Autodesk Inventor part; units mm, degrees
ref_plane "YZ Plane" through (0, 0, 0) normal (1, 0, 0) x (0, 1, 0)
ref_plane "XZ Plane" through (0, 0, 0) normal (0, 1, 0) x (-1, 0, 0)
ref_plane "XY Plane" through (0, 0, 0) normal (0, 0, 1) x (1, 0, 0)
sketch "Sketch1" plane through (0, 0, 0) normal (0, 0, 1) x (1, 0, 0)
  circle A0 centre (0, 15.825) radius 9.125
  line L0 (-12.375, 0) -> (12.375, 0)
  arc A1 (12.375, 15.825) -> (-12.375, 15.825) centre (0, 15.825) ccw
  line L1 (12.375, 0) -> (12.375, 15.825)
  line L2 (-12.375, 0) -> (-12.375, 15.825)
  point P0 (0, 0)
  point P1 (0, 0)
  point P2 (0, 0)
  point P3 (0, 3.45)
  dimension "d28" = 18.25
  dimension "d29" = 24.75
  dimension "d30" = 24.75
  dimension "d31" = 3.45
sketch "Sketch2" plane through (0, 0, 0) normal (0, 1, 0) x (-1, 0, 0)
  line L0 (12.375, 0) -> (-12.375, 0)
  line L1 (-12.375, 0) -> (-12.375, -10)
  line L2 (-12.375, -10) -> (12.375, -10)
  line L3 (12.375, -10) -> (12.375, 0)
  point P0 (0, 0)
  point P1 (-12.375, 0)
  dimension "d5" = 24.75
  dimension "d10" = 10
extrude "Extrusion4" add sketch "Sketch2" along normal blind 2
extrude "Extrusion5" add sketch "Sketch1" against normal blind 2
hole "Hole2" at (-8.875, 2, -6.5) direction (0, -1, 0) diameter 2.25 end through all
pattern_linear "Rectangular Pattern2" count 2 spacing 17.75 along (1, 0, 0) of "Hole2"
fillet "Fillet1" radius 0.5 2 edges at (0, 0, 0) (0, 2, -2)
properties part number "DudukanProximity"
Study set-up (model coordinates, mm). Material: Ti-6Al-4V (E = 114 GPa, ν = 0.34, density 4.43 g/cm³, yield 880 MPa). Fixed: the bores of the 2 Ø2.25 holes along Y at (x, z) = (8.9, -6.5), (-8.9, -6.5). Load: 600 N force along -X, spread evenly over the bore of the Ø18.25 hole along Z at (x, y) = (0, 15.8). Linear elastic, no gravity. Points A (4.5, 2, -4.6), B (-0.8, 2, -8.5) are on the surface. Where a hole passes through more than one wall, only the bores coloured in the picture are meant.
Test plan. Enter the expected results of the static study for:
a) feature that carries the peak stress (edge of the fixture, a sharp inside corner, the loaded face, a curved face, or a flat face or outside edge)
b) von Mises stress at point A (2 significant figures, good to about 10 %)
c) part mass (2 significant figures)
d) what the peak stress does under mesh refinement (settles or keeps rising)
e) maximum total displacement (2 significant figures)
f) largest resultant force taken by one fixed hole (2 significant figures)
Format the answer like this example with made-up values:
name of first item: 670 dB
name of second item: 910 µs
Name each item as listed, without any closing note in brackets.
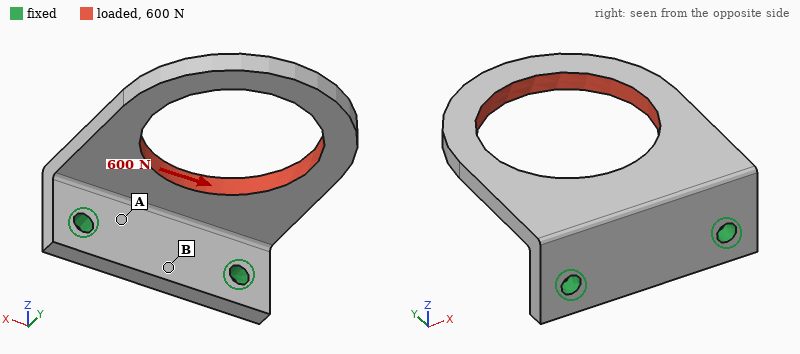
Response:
feature that carries the peak stress: edge of the fixture
von Mises stress at point A: 93 MPa
part mass: 5.0 g
what the peak stress does under mesh refinement: keeps rising
maximum total displacement: 0.15 mm
largest resultant force taken by one fixed hole: 580 N
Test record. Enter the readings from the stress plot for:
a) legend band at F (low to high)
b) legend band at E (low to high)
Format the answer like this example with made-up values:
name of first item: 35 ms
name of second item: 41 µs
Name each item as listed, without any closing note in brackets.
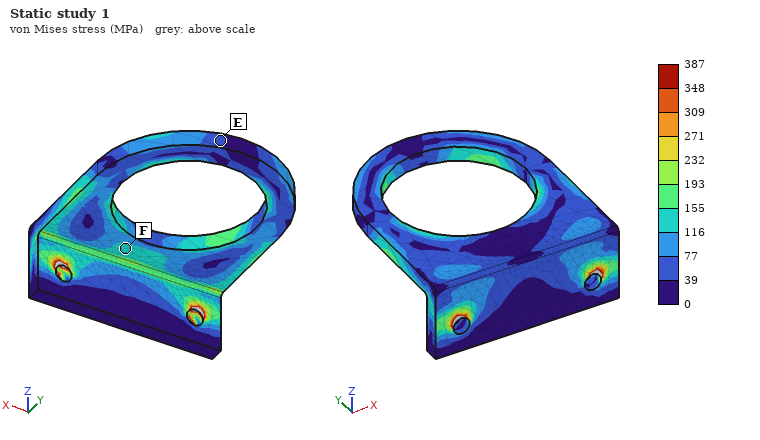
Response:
legend band at F: 116 to 155 MPa
legend band at E: 39 to 77 MPa
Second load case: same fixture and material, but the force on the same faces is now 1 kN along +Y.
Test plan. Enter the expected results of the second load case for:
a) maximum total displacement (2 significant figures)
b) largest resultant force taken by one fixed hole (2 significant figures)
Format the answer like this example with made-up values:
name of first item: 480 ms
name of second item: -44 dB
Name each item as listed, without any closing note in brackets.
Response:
maximum total displacement: 0.25 mm
largest resultant force taken by one fixed hole: 500 N
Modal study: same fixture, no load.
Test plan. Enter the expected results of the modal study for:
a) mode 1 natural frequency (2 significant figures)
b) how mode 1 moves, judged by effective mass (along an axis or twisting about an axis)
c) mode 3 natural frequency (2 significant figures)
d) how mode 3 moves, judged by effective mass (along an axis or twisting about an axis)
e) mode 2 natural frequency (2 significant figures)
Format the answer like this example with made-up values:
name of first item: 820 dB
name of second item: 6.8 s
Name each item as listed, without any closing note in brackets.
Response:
mode 1 natural frequency: 2200 Hz
how mode 1 moves, judged by effective mass: along Z
mode 3 natural frequency: 8400 Hz
how mode 3 moves, judged by effective mass: along X
mode 2 natural frequency: 5600 Hz
